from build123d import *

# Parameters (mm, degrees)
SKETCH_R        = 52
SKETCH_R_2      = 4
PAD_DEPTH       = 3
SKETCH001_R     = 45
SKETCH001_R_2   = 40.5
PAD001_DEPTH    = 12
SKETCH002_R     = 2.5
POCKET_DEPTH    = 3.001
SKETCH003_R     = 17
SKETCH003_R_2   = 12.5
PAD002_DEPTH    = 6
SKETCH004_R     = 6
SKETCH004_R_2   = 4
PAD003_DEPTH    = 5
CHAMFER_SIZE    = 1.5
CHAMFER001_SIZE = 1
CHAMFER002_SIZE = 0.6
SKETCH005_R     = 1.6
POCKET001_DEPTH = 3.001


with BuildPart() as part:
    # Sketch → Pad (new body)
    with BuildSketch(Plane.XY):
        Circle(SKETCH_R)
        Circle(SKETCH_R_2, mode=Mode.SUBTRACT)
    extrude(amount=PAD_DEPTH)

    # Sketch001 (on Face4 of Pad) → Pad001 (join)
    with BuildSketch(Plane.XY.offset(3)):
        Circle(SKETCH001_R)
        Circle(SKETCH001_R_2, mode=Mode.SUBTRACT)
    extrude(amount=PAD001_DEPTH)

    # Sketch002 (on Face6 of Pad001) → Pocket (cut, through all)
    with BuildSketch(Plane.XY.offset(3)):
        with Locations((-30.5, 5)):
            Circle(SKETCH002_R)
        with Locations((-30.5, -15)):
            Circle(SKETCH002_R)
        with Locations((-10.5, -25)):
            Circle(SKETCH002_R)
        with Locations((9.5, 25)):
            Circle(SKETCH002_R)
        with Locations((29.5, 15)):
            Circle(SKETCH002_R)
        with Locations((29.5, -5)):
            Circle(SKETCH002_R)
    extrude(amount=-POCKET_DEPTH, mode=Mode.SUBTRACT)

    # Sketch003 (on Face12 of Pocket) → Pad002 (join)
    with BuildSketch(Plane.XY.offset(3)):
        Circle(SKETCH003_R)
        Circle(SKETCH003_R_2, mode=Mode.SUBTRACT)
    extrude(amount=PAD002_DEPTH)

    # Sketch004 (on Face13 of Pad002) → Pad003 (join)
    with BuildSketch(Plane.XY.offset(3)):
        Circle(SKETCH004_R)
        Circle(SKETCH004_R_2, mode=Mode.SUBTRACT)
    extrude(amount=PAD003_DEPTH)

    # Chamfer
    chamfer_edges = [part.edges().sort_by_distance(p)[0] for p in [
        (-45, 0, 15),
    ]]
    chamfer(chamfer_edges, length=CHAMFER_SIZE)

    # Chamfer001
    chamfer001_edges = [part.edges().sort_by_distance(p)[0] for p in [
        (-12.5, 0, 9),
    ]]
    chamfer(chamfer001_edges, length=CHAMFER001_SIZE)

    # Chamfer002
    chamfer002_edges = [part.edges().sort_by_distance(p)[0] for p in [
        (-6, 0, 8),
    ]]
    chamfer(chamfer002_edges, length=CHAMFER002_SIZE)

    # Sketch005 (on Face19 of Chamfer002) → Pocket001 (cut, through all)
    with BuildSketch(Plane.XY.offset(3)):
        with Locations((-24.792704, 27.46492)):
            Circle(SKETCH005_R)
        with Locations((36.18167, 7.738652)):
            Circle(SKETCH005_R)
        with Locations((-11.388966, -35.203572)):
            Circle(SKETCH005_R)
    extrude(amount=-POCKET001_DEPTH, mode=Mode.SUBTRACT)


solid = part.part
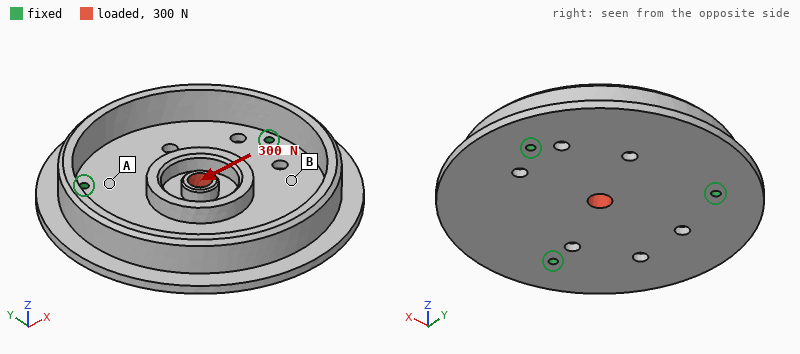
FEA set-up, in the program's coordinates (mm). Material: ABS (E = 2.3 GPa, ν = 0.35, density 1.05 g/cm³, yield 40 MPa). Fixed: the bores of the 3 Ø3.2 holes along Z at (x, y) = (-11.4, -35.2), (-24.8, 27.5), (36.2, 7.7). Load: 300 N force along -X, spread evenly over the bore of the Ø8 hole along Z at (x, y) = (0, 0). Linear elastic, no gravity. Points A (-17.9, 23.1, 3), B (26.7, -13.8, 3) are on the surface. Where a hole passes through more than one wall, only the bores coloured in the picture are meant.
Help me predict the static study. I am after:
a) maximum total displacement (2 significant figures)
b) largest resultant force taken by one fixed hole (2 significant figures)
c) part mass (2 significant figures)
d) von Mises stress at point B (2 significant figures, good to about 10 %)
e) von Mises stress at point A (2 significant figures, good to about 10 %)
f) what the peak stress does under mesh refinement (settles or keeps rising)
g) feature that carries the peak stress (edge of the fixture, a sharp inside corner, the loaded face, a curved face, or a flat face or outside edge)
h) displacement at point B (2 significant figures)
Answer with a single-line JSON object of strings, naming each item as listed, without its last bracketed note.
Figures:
{"maximum total displacement": "0.13 mm", "largest resultant force taken by one fixed hole": "110 N", "part mass": "44 g", "von Mises stress at point B": "0.80 MPa", "von Mises stress at point A": "2.1 MPa", "what the peak stress does under mesh refinement": "keeps rising", "feature that carries the peak stress": "edge of the fixture", "displacement at point B": "0.036 mm"}
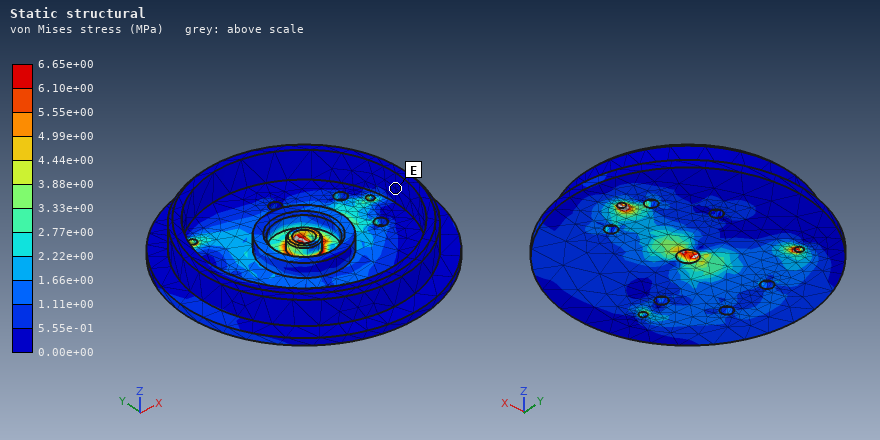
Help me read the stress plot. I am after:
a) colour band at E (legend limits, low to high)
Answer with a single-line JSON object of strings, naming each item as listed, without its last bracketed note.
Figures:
{"colour band at E": "0.00e+00 to 5.55e-01 MPa"}
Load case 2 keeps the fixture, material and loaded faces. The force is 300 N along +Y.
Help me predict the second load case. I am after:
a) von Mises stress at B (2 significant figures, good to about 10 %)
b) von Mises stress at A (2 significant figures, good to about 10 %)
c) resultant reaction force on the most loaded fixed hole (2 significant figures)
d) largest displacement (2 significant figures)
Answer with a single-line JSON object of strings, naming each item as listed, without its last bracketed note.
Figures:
{"von Mises stress at B": "0.66 MPa", "von Mises stress at A": "1.7 MPa", "resultant reaction force on the most loaded fixed hole": "110 N", "largest displacement": "0.13 mm"}
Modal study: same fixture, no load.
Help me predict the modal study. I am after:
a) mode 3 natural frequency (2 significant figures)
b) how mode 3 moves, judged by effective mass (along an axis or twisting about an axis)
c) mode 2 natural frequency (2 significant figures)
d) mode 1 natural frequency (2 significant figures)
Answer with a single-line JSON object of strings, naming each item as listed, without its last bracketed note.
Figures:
{"mode 3 natural frequency": "1300 Hz", "how mode 3 moves, judged by effective mass": "along Z", "mode 2 natural frequency": "780 Hz", "mode 1 natural frequency": "780 Hz"}
